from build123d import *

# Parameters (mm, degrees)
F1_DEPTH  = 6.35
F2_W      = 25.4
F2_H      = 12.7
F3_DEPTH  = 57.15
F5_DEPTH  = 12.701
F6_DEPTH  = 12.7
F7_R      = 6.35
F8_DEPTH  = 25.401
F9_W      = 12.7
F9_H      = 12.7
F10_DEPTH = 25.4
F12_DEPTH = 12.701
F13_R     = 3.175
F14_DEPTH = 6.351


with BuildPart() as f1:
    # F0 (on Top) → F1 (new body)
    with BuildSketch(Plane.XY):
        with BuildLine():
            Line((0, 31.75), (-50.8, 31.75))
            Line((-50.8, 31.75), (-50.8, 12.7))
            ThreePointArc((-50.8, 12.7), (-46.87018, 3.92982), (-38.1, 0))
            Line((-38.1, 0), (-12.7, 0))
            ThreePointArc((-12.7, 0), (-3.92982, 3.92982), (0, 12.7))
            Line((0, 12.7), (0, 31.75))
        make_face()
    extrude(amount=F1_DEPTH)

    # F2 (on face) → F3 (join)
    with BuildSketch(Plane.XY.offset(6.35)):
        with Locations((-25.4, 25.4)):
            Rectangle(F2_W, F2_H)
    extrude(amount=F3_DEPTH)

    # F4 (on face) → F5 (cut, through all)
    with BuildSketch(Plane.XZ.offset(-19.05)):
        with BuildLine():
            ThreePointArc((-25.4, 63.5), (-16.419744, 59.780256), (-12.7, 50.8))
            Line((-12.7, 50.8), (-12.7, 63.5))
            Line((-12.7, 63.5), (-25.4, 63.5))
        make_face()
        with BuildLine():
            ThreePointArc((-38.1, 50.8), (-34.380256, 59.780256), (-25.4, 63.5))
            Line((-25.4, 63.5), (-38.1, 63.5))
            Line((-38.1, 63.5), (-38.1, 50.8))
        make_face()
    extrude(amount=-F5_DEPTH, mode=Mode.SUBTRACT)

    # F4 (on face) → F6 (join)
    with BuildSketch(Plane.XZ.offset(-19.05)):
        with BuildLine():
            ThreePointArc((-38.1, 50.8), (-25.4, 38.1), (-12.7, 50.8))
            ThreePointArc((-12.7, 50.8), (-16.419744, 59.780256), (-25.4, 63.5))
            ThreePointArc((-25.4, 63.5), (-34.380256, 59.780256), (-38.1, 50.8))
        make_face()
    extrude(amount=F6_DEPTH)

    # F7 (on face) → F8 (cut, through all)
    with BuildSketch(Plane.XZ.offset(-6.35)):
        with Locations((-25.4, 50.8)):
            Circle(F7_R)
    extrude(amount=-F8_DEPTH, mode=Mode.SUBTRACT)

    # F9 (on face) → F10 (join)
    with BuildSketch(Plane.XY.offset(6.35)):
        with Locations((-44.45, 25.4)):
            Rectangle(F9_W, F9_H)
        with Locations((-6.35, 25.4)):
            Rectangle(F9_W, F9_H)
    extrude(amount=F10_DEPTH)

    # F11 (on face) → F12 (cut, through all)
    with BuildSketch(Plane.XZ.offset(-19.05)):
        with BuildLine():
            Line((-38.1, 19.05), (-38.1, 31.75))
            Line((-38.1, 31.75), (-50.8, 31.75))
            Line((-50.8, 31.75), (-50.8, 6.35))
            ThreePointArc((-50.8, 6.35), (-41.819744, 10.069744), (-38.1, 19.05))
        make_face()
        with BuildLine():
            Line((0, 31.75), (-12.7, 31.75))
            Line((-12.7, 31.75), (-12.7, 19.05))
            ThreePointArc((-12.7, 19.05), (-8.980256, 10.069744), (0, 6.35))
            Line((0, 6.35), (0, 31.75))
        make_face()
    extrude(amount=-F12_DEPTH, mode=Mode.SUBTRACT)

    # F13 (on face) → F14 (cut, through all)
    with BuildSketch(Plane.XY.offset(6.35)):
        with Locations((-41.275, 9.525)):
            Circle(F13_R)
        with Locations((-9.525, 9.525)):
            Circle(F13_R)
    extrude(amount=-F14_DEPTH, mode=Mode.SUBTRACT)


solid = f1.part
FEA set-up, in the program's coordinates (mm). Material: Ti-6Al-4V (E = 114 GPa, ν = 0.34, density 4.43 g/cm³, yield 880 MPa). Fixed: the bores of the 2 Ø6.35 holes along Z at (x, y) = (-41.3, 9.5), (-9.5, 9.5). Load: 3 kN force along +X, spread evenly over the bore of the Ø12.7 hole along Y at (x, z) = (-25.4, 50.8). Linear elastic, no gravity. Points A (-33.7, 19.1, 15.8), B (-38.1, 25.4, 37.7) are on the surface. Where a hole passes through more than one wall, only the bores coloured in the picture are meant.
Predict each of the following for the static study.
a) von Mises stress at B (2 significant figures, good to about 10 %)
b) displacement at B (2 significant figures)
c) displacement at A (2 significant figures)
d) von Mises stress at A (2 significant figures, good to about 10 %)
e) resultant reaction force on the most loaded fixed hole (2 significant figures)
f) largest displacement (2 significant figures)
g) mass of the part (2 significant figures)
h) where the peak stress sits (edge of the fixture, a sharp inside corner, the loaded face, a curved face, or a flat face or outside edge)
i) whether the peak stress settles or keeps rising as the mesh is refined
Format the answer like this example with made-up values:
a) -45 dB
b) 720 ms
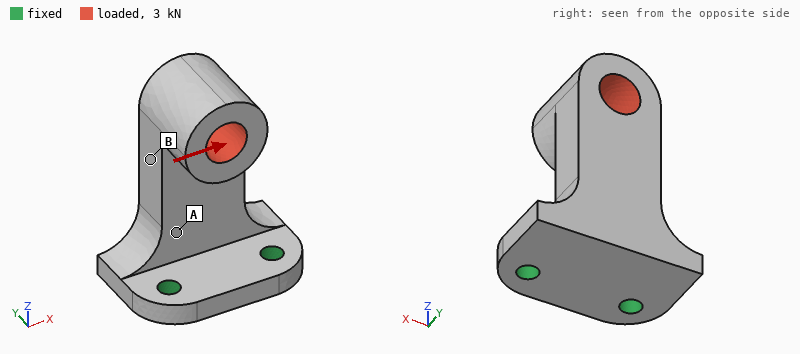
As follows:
a) 37 MPa
b) 0.11 mm
c) 0.039 mm
d) 86 MPa
e) 4.6 kN
f) 0.23 mm
g) 140 g
h) edge of the fixture
i) keeps rising
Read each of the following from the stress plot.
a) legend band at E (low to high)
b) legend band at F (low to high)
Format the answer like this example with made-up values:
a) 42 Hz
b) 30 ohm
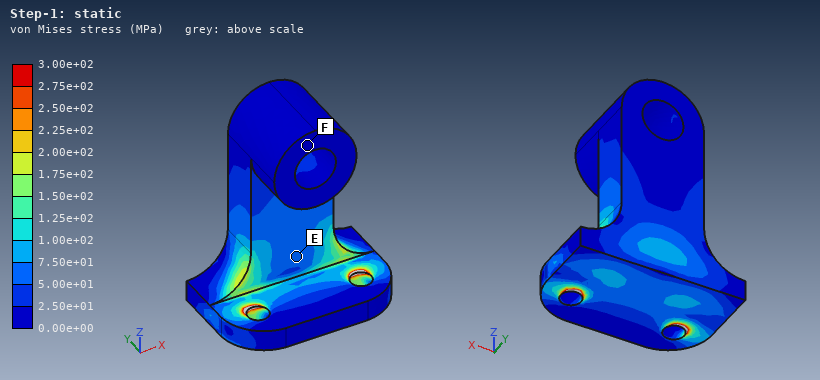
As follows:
a) 5.00e+01 to 7.50e+01 MPa
b) 0.00e+00 to 2.50e+01 MPa
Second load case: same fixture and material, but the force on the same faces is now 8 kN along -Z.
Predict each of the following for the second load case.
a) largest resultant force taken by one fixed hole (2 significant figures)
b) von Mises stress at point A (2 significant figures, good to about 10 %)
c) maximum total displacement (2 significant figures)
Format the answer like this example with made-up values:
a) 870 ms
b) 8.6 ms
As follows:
a) 4.0 kN
b) 90 MPa
c) 92 µm
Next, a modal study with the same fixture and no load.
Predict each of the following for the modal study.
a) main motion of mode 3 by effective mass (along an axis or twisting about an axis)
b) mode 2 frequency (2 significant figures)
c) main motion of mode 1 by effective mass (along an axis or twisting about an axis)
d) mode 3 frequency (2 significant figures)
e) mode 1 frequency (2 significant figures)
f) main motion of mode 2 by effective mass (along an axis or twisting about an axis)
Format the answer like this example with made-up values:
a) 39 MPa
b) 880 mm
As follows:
a) along Z
b) 2900 Hz
c) along Y
d) 6000 Hz
e) 1200 Hz
f) along X
